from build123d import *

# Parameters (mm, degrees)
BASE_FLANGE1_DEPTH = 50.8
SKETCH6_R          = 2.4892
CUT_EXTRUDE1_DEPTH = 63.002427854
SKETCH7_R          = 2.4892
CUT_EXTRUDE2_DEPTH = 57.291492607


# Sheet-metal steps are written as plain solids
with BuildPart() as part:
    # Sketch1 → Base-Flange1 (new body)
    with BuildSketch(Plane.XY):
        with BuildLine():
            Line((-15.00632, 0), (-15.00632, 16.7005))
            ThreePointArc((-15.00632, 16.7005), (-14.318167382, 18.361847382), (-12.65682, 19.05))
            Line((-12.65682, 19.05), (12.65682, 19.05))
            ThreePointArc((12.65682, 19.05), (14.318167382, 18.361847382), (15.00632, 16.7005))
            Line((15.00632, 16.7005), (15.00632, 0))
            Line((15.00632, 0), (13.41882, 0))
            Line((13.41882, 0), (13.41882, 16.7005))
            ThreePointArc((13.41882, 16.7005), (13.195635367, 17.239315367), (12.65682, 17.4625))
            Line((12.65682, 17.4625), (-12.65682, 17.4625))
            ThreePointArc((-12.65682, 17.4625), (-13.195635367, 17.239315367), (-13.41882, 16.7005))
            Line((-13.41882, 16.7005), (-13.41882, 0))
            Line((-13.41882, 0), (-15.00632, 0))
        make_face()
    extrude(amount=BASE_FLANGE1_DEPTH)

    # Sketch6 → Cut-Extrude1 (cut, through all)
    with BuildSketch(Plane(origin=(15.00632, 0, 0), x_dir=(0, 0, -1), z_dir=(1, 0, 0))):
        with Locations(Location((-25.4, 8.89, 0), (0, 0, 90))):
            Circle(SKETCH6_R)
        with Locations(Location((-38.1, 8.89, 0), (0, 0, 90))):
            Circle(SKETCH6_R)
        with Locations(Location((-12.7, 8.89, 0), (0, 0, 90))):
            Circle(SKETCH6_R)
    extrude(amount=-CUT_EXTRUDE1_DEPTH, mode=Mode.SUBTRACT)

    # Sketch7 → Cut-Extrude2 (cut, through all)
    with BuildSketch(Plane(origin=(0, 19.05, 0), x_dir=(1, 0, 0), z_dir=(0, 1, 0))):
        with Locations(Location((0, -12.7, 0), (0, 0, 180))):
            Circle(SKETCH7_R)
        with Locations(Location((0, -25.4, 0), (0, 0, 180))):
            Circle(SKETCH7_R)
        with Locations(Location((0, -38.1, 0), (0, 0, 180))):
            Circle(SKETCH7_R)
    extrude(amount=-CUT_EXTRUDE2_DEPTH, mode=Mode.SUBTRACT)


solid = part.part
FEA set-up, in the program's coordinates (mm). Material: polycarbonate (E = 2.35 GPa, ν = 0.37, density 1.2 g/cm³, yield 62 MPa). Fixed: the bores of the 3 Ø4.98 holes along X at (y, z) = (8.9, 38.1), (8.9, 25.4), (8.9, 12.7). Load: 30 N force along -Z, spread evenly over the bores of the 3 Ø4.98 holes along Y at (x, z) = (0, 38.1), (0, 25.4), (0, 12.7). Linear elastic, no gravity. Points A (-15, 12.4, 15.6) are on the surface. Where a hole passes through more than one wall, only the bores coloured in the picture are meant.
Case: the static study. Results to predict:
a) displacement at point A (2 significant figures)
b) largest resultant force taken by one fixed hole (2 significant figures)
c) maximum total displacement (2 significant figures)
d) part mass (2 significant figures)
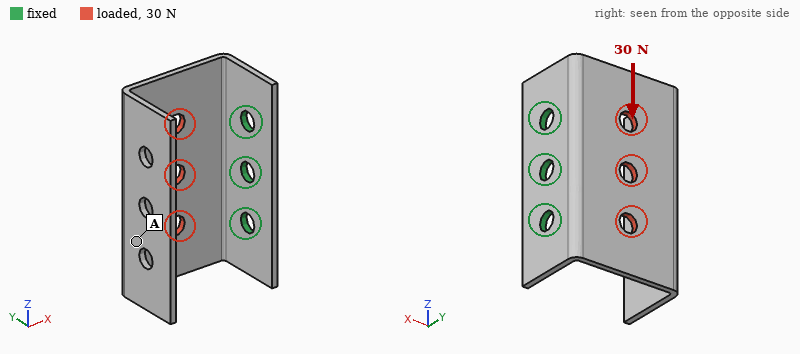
0.35 mm
19 N
0.58 mm
5.8 g
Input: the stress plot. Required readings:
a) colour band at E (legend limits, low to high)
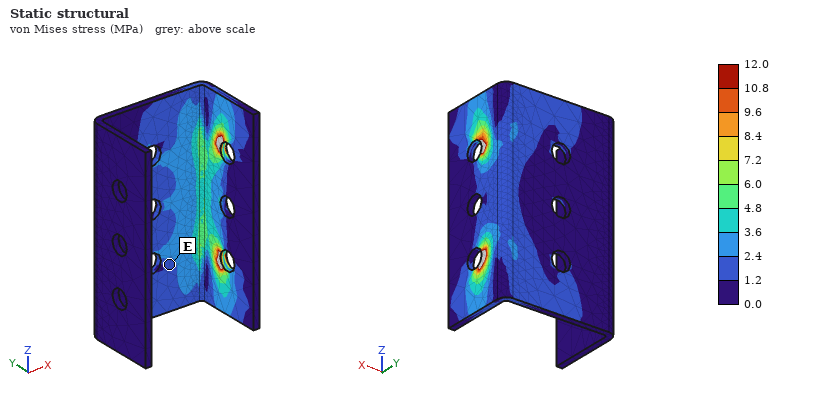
1.2 to 2.4 MPa
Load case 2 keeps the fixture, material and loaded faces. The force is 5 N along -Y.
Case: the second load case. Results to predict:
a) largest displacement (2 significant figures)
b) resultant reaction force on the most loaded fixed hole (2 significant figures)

0.73 mm
1.9 N
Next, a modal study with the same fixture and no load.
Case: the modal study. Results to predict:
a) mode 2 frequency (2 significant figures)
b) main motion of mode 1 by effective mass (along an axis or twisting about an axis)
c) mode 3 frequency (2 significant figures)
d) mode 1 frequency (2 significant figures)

310 Hz
along Y
610 Hz
170 Hz
